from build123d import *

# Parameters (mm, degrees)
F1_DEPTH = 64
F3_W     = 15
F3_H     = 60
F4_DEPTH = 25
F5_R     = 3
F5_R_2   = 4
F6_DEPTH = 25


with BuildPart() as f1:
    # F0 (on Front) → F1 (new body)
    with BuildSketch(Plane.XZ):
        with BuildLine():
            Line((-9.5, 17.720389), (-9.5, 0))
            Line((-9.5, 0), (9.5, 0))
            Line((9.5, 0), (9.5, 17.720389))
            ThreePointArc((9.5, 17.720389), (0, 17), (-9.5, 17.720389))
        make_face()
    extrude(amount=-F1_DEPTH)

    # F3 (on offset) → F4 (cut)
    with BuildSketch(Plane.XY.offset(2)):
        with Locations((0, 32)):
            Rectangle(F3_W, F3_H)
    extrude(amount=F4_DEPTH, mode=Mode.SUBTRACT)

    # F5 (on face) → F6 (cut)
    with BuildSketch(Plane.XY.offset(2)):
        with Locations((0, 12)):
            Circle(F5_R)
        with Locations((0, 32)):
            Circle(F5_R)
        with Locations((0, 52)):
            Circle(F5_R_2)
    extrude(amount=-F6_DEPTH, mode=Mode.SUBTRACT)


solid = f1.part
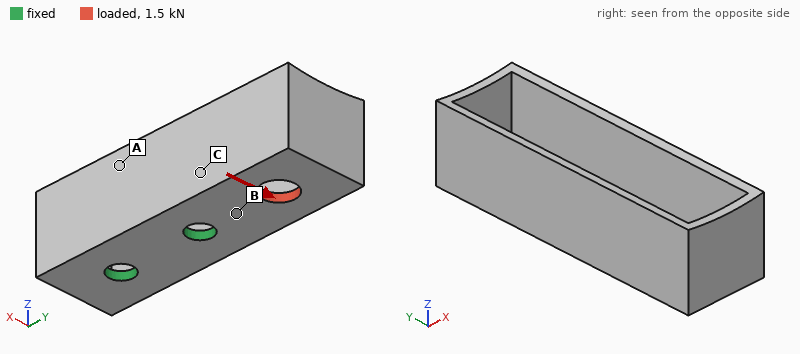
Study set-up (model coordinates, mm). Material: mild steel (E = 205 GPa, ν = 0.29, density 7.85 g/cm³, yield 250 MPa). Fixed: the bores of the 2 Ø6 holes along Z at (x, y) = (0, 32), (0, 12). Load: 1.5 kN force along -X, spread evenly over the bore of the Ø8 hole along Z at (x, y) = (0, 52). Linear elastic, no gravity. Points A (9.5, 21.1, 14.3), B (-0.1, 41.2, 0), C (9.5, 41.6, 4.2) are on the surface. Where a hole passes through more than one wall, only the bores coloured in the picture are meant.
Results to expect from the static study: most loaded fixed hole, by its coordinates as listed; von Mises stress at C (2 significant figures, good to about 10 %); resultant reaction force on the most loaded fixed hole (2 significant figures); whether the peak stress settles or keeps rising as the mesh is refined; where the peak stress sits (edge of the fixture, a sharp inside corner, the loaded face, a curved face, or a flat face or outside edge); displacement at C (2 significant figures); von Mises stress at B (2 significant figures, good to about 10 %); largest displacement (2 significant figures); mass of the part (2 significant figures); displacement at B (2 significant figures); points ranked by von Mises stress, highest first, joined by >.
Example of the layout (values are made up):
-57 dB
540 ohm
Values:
(0, 32)
53 MPa
2.3 kN
keeps rising
edge of the fixture
16 µm
95 MPa
66 µm
56 g
11 µm
B > C > A
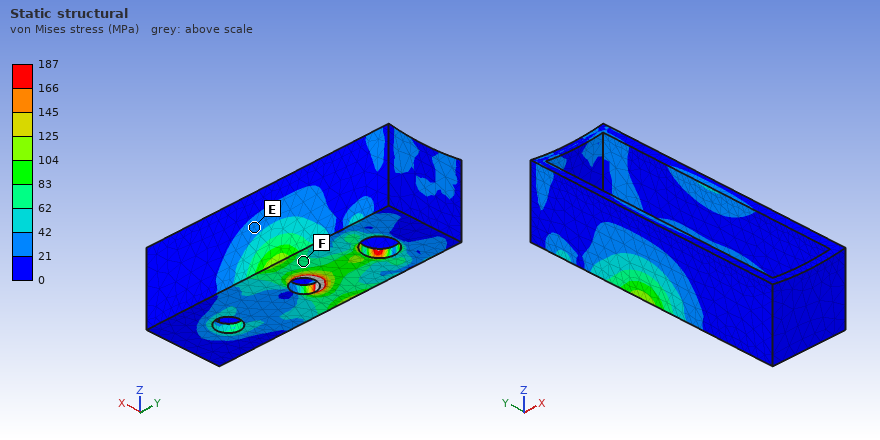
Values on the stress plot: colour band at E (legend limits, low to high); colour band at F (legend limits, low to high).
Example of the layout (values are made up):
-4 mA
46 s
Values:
21 to 42 MPa
62 to 83 MPa
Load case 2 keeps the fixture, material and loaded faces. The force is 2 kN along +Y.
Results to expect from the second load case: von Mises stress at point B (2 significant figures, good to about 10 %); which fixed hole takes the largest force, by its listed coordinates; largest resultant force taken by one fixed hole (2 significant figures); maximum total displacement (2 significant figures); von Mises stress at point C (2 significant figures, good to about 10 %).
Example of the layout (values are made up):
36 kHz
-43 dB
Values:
59 MPa
(0, 32)
1.7 kN
10.0 µm
21 MPa
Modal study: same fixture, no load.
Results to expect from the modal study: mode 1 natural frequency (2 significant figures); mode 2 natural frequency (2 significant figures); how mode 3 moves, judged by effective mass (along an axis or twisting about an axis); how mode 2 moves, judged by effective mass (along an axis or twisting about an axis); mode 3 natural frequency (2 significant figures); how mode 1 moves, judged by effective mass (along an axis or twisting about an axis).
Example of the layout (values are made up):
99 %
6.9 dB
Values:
2800 Hz
3700 Hz
along X
along Z
4700 Hz
along X
